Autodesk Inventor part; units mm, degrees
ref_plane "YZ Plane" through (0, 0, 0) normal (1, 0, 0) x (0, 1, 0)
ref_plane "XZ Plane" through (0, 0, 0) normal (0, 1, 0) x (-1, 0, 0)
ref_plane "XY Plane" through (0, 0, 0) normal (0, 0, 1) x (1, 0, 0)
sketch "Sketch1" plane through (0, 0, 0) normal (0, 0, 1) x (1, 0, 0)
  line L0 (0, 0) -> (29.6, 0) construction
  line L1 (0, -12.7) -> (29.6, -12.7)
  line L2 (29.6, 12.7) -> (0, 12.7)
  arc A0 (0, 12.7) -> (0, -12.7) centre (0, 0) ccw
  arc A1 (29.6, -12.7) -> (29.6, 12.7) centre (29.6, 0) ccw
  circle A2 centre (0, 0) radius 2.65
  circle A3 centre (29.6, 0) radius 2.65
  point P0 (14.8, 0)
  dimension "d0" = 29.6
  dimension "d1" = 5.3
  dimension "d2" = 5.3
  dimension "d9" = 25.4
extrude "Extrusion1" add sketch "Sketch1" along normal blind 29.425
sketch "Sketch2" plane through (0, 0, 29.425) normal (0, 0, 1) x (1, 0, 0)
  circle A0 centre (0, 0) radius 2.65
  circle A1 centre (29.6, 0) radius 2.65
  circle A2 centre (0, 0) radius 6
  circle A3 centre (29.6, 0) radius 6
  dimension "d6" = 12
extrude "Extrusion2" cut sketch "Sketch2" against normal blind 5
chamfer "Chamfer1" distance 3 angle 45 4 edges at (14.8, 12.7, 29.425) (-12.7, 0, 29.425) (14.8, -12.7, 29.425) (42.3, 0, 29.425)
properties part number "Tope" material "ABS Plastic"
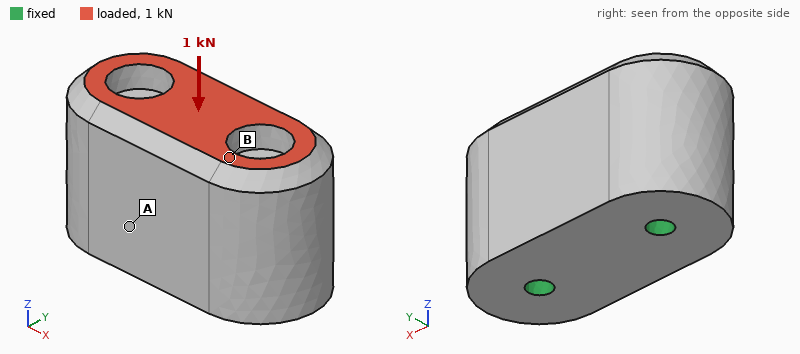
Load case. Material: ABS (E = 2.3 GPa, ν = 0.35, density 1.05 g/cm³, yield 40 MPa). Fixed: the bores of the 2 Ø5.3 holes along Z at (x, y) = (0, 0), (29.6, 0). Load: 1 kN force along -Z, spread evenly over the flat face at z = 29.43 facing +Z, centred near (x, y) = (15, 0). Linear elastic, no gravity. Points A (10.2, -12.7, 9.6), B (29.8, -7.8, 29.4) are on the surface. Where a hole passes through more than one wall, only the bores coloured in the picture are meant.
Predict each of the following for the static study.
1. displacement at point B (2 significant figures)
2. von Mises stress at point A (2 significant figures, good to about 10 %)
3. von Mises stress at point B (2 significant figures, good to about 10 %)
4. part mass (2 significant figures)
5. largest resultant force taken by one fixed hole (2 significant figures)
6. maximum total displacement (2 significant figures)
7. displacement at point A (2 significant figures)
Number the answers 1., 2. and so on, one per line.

1. 10 µm
2. 0.43 MPa
3. 1.1 MPa
4. 36 g
5. 510 N
6. 14 µm
7. 7.6 µm
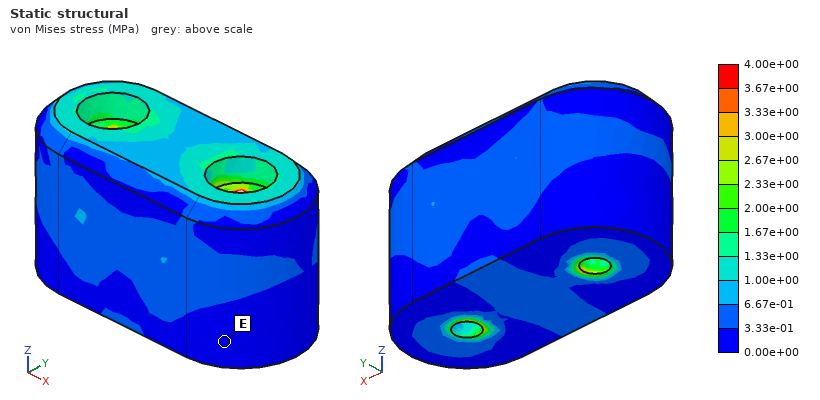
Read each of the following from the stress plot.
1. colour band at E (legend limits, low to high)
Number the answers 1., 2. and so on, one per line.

1. 0.00e+00 to 3.33e-01 MPa
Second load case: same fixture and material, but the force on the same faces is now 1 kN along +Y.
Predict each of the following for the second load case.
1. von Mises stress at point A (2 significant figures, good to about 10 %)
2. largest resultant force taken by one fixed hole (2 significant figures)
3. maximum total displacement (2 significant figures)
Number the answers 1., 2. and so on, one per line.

1. 1.2 MPa
2. 500 N
3. 52 µm
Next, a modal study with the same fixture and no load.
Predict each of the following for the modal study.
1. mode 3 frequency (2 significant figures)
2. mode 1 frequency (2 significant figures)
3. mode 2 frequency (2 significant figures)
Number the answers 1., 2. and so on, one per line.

1. 11 kHz
2. 9400 Hz
3. 11 kHz
